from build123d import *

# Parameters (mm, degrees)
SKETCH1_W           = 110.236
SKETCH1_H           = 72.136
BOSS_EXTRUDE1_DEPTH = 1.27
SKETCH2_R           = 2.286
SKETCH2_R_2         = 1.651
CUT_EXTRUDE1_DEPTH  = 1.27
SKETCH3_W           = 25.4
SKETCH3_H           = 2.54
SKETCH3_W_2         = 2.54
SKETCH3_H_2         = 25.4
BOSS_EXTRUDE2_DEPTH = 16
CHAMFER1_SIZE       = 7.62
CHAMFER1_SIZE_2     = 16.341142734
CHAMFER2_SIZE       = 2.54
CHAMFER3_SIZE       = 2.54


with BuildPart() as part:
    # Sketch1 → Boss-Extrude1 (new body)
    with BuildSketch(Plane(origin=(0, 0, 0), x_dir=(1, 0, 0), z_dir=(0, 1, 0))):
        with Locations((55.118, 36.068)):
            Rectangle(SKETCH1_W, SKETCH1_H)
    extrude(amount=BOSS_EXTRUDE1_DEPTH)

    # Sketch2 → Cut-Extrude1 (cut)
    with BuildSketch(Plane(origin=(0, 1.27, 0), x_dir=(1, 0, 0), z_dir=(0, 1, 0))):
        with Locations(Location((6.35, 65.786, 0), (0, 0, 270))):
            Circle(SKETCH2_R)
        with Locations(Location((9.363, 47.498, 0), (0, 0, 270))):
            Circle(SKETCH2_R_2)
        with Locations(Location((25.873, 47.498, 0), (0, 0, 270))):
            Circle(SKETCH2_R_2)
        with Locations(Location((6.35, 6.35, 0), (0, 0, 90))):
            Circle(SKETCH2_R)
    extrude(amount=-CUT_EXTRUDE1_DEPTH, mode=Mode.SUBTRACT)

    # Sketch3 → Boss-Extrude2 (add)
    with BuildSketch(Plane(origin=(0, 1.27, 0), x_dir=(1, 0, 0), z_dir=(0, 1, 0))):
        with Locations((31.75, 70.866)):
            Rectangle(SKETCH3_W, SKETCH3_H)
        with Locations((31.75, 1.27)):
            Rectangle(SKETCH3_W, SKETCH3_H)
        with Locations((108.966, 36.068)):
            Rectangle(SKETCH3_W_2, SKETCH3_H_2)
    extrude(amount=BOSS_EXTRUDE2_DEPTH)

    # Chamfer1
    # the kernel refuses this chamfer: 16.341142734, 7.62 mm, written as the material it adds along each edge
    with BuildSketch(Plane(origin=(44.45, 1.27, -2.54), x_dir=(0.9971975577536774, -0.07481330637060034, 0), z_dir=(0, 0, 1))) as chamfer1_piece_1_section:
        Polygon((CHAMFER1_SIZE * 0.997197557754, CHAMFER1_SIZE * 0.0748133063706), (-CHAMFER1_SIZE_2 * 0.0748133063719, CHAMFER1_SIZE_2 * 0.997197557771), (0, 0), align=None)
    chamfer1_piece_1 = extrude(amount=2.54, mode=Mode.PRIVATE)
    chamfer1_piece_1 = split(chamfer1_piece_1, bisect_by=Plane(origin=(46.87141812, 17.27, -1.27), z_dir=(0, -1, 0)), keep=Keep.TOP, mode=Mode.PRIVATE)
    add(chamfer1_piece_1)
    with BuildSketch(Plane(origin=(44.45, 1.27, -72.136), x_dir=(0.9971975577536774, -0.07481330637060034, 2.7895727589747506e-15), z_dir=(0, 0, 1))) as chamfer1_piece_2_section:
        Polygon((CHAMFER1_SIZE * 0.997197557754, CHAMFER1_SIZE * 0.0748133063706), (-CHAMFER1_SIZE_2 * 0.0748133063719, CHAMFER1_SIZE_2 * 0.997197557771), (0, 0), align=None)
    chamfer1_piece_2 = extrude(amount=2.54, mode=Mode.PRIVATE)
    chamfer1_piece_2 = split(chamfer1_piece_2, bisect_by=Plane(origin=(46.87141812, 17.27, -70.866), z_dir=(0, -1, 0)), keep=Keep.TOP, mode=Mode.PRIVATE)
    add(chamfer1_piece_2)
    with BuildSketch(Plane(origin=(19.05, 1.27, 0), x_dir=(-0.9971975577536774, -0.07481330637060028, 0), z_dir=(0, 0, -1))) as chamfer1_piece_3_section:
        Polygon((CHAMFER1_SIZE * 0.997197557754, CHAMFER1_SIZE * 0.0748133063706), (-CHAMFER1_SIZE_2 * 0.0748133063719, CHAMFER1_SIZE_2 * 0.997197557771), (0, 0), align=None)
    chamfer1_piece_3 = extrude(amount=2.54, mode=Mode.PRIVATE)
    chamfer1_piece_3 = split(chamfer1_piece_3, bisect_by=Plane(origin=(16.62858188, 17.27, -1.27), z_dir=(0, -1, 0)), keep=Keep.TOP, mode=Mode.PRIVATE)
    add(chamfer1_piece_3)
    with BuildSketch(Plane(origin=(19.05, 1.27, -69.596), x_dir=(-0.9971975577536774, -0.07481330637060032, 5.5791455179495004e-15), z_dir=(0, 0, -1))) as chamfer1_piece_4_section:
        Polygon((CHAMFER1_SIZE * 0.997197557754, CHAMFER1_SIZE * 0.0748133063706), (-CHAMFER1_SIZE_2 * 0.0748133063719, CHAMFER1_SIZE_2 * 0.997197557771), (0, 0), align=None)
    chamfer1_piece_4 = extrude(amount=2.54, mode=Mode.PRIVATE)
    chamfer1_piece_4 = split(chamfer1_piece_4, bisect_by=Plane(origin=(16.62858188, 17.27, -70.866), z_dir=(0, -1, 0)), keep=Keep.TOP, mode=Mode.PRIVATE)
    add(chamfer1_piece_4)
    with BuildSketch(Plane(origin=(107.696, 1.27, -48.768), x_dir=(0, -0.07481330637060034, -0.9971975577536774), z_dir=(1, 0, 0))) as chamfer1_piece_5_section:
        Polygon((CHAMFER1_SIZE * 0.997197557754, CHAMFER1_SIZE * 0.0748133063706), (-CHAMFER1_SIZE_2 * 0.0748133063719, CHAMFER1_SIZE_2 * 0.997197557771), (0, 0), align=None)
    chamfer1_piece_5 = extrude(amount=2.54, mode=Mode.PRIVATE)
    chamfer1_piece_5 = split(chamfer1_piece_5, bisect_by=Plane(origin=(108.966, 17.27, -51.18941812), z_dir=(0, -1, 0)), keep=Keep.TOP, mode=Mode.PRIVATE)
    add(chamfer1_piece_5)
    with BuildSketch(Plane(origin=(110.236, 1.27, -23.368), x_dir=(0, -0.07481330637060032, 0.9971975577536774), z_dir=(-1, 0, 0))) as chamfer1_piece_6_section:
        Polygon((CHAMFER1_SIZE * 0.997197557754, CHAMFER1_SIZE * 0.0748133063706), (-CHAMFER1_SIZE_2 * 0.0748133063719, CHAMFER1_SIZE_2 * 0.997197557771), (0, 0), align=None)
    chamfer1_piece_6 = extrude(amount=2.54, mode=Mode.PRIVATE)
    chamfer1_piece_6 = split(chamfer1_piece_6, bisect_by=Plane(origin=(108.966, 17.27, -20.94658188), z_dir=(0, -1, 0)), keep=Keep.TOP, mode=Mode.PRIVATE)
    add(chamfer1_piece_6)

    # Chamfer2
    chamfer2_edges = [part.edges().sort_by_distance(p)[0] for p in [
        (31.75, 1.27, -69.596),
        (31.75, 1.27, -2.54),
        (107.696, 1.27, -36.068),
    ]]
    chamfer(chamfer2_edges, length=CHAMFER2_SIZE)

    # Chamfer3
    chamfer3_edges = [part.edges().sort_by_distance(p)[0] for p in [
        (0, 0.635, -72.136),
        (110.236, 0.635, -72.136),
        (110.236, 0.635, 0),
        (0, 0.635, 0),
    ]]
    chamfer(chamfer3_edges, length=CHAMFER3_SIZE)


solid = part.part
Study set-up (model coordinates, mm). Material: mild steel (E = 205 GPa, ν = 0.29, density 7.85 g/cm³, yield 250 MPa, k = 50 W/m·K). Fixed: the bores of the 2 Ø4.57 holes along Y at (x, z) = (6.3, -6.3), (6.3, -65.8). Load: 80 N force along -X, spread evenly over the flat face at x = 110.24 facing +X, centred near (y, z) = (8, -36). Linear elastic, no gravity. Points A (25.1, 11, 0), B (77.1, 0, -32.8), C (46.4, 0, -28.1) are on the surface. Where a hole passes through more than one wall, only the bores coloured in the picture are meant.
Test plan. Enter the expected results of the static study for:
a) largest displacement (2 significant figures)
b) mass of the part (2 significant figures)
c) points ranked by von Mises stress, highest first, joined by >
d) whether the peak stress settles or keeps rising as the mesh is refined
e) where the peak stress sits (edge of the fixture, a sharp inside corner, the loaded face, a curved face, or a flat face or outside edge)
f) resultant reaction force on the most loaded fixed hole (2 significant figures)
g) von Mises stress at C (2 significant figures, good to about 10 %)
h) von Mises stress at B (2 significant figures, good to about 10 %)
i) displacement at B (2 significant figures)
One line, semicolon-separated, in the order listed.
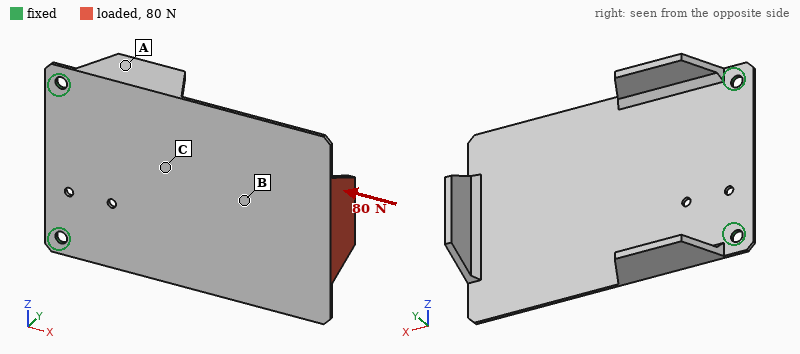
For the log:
0.74 mm; 110 g; B > C > A; keeps rising; edge of the fixture; 40 N; 14 MPa; 25 MPa; 0.28 mm
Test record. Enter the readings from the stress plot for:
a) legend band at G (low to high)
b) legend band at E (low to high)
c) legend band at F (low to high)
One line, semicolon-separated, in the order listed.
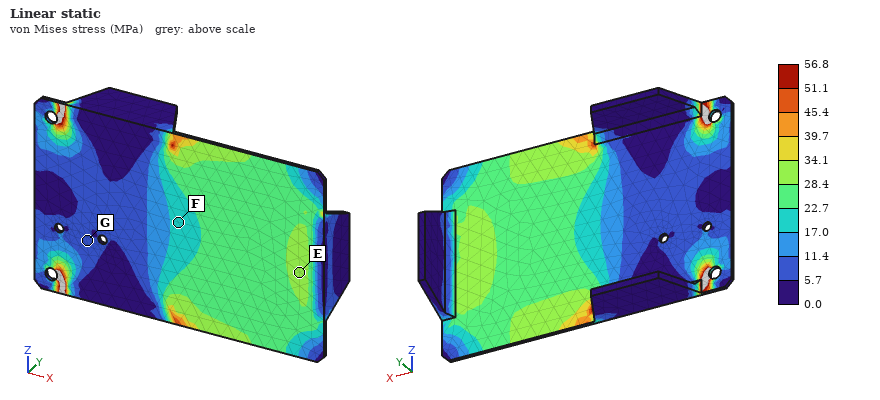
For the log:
5.7 to 11.4 MPa; 28.4 to 34.1 MPa; 17.0 to 22.7 MPa
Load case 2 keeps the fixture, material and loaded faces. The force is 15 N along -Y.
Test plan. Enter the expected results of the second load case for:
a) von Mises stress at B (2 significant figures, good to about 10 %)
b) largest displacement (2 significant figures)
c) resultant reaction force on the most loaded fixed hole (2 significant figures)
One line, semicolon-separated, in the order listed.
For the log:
24 MPa; 1.2 mm; 28 N
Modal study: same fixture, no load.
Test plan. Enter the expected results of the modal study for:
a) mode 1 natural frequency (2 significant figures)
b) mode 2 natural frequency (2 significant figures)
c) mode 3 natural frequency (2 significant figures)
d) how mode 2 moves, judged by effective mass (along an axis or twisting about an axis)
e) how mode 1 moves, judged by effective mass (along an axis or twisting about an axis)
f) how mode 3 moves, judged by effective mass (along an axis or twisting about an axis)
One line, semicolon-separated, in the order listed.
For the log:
100 Hz; 350 Hz; 480 Hz; twisting about X; along Y; along Y
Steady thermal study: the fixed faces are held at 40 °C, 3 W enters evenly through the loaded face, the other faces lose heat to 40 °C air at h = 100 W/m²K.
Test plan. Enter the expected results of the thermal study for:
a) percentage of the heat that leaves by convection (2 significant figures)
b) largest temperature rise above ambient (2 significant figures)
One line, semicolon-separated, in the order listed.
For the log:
100 %; 13 K
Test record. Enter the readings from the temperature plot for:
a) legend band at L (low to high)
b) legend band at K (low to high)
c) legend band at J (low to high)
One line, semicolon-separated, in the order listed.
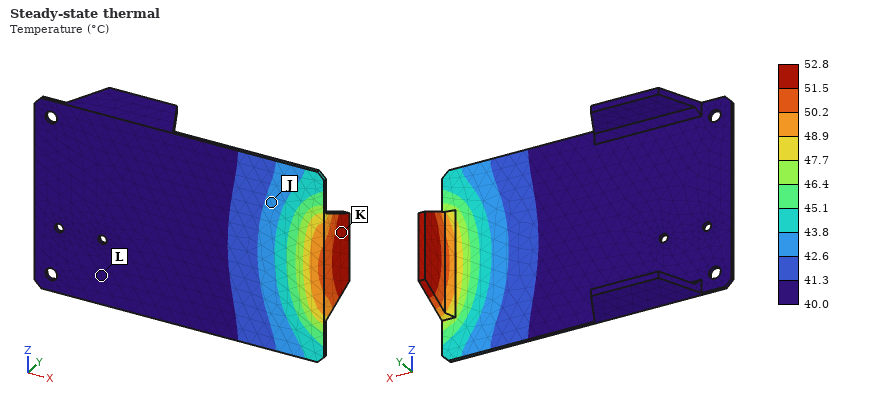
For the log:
40.0 to 41.3 °C; 51.5 to 52.8 °C; 42.6 to 43.8 °C
